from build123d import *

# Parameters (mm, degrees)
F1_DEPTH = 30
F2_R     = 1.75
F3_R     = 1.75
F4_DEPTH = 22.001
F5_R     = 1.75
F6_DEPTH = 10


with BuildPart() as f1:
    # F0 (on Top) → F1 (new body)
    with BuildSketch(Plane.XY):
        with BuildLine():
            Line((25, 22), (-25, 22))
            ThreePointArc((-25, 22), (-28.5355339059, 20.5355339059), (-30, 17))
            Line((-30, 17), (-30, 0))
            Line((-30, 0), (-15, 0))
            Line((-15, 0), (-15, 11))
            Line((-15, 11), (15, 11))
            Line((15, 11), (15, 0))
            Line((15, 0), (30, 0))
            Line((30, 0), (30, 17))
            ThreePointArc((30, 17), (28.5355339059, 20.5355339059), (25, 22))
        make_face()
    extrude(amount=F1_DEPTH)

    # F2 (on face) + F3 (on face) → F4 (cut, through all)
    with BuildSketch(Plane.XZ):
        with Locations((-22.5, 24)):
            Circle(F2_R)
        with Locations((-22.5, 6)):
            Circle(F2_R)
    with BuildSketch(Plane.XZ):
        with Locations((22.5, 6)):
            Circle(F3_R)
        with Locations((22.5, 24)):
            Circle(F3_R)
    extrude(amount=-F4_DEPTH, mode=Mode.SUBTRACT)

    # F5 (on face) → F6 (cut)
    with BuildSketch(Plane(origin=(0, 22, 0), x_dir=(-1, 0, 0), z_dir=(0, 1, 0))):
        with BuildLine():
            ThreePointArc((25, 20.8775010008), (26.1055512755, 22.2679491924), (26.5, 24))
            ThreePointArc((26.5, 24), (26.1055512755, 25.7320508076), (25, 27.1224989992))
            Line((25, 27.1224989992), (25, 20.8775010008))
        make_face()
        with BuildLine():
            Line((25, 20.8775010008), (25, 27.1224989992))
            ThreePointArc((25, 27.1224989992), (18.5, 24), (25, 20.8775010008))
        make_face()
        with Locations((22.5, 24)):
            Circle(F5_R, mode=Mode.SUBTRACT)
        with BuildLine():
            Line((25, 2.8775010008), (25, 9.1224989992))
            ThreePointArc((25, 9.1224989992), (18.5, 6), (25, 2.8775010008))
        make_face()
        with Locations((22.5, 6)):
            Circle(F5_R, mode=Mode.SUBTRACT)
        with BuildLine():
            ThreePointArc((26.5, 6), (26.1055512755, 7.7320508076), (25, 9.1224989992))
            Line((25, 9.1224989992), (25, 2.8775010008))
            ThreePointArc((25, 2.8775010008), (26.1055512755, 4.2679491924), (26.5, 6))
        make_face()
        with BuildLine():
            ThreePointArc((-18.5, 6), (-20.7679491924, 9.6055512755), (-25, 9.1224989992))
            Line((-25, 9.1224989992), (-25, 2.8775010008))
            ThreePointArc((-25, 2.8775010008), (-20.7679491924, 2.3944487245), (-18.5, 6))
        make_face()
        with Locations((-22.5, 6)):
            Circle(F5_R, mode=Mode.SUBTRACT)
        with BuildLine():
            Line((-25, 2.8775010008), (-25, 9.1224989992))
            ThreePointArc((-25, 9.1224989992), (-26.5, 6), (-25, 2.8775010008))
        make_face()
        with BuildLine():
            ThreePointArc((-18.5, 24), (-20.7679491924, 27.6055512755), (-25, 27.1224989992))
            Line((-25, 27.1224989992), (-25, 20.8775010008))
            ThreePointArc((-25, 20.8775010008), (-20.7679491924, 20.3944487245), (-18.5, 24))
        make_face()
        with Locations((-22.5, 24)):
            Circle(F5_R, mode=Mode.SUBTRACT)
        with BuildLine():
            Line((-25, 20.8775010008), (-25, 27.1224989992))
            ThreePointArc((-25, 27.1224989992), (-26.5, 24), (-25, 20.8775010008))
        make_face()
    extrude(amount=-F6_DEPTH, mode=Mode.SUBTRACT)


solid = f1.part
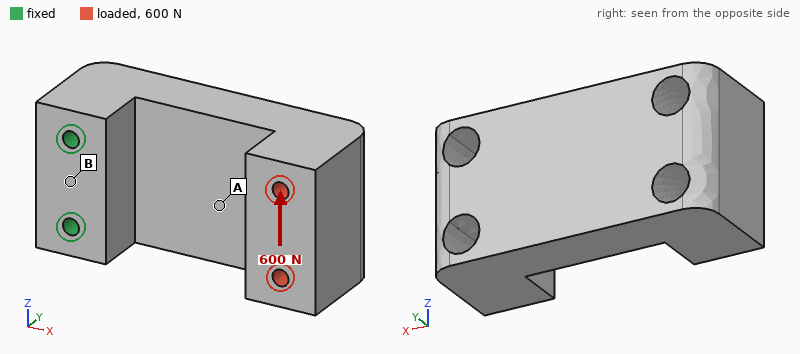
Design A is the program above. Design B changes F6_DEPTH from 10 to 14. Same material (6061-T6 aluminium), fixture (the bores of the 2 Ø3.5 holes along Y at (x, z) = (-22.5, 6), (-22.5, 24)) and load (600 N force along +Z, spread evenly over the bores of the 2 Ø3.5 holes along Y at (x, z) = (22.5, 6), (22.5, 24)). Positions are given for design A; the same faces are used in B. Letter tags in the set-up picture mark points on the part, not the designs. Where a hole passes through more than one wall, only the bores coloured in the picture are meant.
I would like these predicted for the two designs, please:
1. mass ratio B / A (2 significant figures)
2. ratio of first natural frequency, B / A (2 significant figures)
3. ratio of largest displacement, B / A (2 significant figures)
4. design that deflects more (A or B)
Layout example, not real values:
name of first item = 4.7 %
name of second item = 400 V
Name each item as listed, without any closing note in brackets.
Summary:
mass ratio B / A = 0.98
ratio of first natural frequency, B / A = 0.89
ratio of largest displacement, B / A = 1.3
design that deflects more = B
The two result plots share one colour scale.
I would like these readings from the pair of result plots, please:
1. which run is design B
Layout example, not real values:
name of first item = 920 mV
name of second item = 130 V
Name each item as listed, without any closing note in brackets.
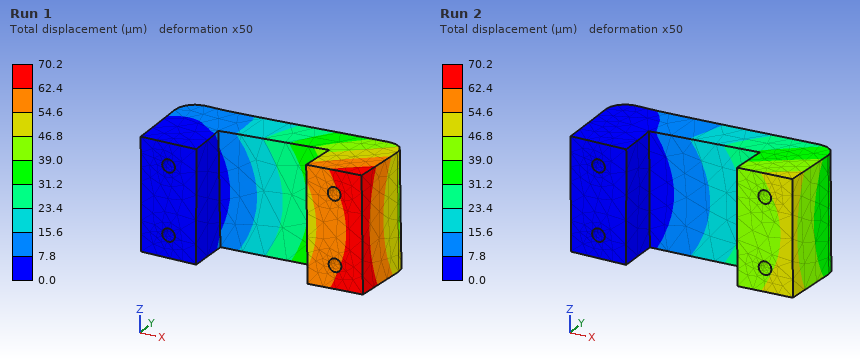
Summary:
which run is design B = Run 1
